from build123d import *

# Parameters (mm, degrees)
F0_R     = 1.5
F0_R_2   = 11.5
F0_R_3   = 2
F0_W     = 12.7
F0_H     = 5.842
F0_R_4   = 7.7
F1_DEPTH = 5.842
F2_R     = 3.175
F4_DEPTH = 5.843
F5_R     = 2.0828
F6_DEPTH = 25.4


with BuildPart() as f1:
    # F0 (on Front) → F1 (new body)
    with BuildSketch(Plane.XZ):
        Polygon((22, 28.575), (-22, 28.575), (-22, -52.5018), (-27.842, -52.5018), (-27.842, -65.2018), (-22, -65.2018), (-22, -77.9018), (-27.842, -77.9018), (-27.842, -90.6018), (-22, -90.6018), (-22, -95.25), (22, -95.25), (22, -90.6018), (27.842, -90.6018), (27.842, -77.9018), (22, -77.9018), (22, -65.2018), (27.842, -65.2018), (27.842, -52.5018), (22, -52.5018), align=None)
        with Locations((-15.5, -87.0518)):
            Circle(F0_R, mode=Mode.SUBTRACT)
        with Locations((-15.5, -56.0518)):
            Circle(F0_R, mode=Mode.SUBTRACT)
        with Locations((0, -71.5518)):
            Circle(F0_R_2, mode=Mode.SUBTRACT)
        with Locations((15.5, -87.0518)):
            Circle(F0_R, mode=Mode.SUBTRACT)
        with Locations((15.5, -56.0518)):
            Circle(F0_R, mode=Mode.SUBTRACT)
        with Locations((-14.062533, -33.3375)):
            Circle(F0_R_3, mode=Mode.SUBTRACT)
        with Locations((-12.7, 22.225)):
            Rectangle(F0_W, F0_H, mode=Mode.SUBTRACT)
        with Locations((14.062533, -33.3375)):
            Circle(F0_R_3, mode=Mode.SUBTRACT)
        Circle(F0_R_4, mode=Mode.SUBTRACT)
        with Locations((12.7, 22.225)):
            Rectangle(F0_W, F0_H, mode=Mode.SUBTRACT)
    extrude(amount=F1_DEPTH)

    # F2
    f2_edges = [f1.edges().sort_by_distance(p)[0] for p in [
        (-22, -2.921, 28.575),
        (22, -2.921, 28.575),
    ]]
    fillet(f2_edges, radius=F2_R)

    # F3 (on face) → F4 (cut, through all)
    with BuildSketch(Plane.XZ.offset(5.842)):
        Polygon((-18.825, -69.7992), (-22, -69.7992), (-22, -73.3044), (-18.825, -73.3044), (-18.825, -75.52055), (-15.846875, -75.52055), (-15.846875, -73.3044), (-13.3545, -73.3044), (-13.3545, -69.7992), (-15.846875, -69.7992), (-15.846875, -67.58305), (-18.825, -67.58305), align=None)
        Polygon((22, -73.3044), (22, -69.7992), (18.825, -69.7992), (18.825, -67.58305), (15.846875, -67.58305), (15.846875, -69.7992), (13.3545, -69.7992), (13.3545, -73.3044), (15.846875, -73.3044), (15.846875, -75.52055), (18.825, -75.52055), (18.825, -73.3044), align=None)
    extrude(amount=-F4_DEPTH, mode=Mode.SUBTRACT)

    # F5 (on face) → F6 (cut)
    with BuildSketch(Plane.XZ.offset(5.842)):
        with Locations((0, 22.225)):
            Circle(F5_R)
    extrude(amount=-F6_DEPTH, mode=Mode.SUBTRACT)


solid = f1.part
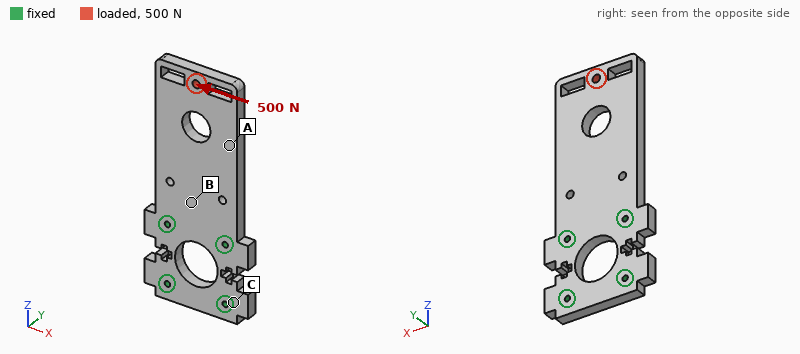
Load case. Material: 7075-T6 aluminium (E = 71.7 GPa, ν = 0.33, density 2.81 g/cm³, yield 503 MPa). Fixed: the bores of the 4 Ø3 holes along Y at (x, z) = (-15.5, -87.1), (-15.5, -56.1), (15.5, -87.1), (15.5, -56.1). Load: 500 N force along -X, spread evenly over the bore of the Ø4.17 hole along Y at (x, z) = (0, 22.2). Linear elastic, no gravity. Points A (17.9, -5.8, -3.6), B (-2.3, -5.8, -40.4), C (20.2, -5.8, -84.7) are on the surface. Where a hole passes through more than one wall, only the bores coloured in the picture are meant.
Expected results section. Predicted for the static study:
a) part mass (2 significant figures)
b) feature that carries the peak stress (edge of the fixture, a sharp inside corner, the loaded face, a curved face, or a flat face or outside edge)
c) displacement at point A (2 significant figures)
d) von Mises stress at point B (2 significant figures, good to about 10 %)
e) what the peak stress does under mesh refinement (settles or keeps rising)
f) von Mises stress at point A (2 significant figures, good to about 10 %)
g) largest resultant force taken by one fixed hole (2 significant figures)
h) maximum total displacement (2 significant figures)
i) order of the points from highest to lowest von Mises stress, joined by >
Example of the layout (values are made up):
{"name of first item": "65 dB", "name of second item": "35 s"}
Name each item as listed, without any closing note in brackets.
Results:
{"part mass": "79 g", "feature that carries the peak stress": "edge of the fixture", "displacement at point A": "24 µm", "von Mises stress at point B": "5.1 MPa", "what the peak stress does under mesh refinement": "keeps rising", "von Mises stress at point A": "7.8 MPa", "largest resultant force taken by one fixed hole": "1.2 kN", "maximum total displacement": "47 µm", "order of the points from highest to lowest von Mises stress, joined by >": "A > B > C"}
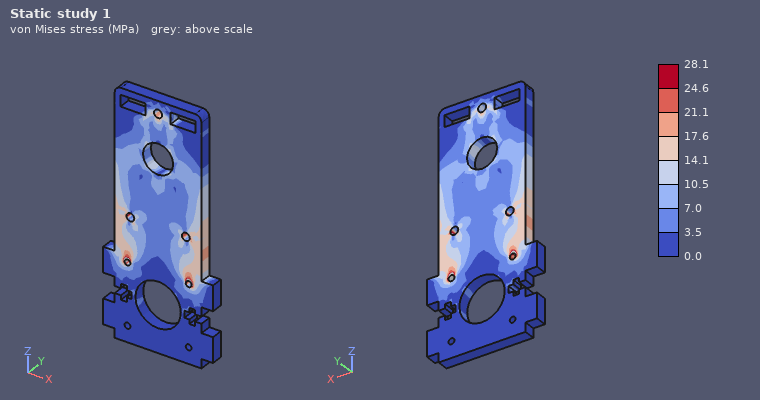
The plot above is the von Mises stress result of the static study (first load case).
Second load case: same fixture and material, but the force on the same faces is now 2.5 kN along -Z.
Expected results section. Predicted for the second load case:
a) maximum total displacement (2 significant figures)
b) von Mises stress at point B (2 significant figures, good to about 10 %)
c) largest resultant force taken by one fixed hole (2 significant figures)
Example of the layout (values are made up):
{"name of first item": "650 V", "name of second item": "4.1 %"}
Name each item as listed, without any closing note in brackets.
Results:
{"maximum total displacement": "24 µm", "von Mises stress at point B": "6.7 MPa", "largest resultant force taken by one fixed hole": "1.2 kN"}
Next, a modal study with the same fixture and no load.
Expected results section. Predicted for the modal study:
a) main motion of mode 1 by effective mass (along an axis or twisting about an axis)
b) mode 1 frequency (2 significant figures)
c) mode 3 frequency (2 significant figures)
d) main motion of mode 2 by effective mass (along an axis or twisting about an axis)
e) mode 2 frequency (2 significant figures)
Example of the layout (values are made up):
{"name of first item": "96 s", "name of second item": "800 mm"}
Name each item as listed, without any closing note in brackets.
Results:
{"main motion of mode 1 by effective mass": "along Y", "mode 1 frequency": "690 Hz", "mode 3 frequency": "3900 Hz", "main motion of mode 2 by effective mass": "twisting about Z", "mode 2 frequency": "2700 Hz"}
